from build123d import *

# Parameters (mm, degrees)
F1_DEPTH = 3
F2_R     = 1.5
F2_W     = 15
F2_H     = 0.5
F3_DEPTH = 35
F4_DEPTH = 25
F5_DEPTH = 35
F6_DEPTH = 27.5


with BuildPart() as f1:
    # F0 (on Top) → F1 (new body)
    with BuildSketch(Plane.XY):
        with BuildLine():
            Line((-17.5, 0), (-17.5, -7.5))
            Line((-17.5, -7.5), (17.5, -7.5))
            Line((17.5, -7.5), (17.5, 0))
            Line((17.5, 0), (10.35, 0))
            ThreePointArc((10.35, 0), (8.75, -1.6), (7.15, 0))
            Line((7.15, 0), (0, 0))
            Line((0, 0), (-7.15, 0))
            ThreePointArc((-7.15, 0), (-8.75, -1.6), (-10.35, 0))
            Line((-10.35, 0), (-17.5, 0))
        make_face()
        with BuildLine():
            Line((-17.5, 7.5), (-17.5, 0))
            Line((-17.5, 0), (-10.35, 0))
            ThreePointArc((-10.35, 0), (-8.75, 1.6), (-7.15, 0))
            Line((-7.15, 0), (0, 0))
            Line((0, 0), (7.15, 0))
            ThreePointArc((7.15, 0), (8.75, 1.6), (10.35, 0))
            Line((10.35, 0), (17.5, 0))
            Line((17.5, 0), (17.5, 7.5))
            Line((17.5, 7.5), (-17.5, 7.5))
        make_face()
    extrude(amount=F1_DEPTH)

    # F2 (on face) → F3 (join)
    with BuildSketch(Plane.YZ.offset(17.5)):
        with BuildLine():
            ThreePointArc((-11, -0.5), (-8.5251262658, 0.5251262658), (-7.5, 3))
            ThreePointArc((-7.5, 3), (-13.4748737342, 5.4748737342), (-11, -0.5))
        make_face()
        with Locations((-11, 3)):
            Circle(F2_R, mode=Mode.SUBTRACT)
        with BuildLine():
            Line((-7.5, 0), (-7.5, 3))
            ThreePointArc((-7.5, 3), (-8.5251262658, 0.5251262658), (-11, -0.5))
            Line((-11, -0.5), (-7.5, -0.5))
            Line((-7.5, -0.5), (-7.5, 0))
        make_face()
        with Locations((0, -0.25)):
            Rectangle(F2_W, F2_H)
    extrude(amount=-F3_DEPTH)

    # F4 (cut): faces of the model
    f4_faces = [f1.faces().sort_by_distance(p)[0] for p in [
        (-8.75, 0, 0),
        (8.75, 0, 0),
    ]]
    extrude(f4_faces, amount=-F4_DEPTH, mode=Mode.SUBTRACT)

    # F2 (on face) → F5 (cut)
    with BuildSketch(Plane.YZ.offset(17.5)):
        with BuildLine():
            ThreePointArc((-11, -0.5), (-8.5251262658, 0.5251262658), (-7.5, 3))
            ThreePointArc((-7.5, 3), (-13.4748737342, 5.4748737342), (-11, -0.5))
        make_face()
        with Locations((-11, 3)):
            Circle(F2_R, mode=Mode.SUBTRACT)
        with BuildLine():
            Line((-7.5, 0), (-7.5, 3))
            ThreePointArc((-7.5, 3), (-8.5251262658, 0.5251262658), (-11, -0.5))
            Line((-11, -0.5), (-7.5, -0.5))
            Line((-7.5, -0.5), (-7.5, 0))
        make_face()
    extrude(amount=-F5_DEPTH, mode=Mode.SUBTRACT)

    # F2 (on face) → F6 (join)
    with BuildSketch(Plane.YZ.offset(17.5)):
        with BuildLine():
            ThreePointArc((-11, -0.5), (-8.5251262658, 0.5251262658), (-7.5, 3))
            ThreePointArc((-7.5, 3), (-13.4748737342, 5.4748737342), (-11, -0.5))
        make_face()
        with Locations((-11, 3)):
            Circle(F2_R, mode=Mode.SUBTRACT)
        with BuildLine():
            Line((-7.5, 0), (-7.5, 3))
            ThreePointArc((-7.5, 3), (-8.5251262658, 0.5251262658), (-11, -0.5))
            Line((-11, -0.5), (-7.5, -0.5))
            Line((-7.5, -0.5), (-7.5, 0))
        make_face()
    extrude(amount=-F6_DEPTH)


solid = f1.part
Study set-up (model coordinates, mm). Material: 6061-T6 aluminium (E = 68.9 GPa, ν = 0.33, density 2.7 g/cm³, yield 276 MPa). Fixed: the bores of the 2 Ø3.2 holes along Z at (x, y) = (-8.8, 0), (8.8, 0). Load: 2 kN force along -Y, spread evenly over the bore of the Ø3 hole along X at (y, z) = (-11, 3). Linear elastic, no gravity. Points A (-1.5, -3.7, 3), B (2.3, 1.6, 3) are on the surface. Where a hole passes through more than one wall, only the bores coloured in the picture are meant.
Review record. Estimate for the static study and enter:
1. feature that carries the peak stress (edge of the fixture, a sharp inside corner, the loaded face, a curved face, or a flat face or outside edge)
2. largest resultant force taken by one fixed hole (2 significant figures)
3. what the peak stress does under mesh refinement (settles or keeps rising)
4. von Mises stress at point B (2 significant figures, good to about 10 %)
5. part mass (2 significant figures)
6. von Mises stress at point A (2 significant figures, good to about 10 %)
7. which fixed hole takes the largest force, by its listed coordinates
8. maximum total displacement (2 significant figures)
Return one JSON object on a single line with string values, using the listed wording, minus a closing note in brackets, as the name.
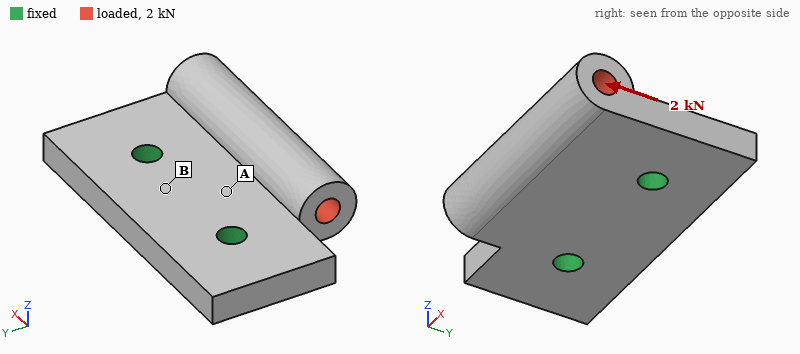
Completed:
{"feature that carries the peak stress": "edge of the fixture", "largest resultant force taken by one fixed hole": "1.4 kN", "what the peak stress does under mesh refinement": "keeps rising", "von Mises stress at point B": "23 MPa", "part mass": "7.3 g", "von Mises stress at point A": "54 MPa", "which fixed hole takes the largest force, by its listed coordinates": "(8.8, 0)", "maximum total displacement": "50 µm"}
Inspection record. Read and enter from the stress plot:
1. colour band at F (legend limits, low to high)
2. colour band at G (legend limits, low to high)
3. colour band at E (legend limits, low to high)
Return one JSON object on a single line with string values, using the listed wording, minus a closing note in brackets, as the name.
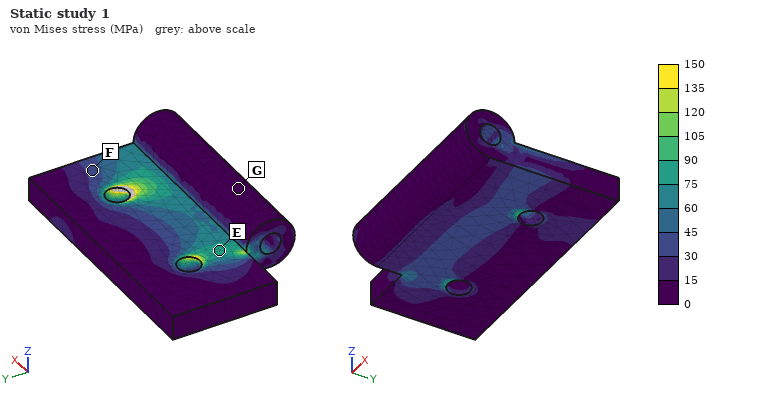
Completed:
{"colour band at F": "30 to 45 MPa", "colour band at G": "0 to 15 MPa", "colour band at E": "75 to 90 MPa"}
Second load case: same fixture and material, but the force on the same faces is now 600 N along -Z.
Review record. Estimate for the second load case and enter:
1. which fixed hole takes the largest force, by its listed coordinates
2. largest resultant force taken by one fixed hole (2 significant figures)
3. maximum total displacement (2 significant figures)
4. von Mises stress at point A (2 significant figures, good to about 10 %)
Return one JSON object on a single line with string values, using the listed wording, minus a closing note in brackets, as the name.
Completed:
{"which fixed hole takes the largest force, by its listed coordinates": "(8.8, 0)", "largest resultant force taken by one fixed hole": "400 N", "maximum total displacement": "65 µm", "von Mises stress at point A": "48 MPa"}
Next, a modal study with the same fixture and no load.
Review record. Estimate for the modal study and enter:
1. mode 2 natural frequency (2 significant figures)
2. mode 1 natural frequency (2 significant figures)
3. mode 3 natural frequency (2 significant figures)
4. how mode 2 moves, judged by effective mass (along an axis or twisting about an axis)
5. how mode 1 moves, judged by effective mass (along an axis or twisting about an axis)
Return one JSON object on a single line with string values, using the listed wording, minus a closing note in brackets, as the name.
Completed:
{"mode 2 natural frequency": "20 kHz", "mode 1 natural frequency": "11 kHz", "mode 3 natural frequency": "33 kHz", "how mode 2 moves, judged by effective mass": "twisting about Y", "how mode 1 moves, judged by effective mass": "along Z"}
